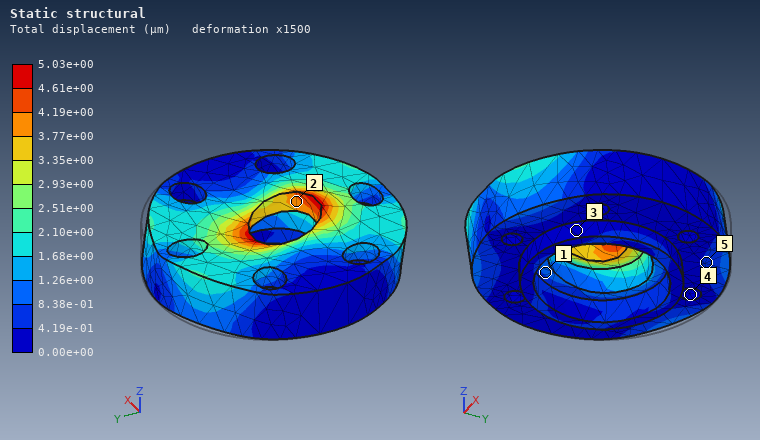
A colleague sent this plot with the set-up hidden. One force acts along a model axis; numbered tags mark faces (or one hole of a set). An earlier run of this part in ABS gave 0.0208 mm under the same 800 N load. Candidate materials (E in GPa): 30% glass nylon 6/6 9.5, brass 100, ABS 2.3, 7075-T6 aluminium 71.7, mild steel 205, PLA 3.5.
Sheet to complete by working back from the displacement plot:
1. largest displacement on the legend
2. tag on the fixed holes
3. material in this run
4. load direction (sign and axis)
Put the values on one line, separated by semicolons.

5.03e+00 µm; 4; 30% glass nylon 6/6; -Y
